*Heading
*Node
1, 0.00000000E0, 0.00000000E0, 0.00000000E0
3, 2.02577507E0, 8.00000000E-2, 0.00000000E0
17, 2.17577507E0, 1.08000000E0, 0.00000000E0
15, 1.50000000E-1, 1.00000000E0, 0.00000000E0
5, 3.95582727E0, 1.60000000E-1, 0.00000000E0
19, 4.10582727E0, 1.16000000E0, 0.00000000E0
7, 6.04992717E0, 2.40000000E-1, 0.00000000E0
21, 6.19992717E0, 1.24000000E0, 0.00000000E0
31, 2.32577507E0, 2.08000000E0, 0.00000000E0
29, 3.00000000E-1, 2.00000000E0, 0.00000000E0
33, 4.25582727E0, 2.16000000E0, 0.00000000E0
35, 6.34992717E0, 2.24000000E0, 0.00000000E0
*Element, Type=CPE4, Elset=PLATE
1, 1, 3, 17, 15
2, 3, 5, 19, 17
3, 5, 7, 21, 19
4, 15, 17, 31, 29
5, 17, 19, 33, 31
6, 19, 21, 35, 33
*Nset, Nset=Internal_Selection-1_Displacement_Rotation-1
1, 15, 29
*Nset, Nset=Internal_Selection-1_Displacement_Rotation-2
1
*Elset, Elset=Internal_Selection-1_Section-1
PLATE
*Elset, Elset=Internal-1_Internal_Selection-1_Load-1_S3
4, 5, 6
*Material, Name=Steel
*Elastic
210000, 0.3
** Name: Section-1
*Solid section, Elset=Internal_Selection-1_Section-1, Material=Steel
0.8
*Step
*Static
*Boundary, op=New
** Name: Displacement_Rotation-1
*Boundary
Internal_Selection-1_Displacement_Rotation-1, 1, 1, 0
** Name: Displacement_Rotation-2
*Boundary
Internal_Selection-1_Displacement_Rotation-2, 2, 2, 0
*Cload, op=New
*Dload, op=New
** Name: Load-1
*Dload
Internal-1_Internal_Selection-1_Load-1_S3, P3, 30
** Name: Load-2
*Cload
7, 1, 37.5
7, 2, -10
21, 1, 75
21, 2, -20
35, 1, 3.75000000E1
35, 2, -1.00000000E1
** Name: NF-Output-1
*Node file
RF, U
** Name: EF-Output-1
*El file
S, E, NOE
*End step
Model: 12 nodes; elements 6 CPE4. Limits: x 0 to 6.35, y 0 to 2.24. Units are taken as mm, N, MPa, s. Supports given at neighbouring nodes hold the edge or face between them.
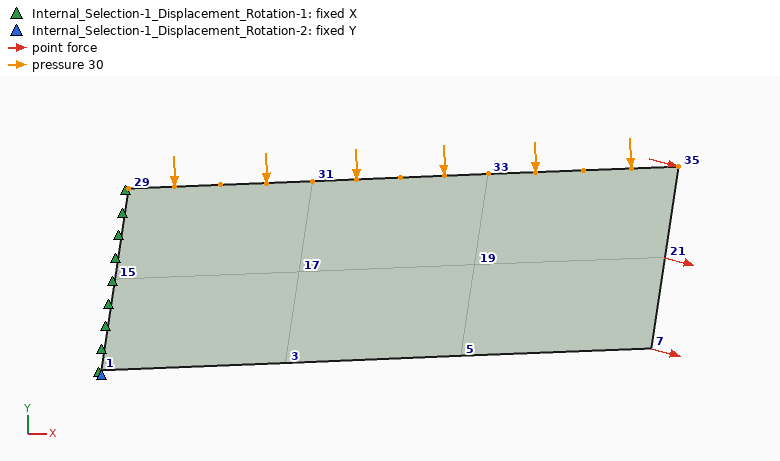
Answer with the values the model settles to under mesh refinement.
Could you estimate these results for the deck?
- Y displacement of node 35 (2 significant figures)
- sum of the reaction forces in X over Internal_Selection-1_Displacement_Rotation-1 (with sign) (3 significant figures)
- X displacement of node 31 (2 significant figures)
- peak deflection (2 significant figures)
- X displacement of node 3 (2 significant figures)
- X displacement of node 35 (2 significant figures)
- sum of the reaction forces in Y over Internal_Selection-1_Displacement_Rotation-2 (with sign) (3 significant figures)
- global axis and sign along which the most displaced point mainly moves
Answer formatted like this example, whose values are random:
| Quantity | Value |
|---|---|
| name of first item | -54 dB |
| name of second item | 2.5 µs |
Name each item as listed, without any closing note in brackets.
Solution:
| Quantity | Value |
|---|---|
| Y displacement of node 35 | -0.077 mm |
| sum of the reaction forces in X over Internal_Selection-1_Displacement_Rotation-1 (with sign) | -156 N |
| X displacement of node 31 | 0.011 mm |
| peak deflection | 0.080 mm |
| X displacement of node 3 | -0.0076 mm |
| X displacement of node 35 | 0.021 mm |
| sum of the reaction forces in Y over Internal_Selection-1_Displacement_Rotation-2 (with sign) | 185 N |
| global axis and sign along which the most displaced point mainly moves | -Y |
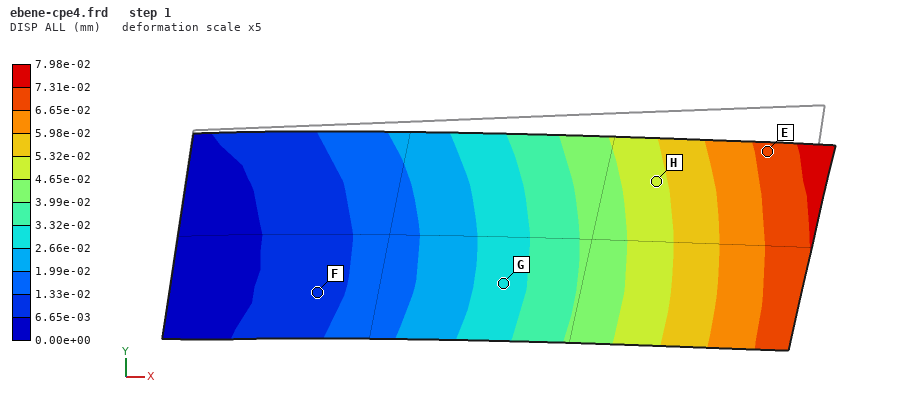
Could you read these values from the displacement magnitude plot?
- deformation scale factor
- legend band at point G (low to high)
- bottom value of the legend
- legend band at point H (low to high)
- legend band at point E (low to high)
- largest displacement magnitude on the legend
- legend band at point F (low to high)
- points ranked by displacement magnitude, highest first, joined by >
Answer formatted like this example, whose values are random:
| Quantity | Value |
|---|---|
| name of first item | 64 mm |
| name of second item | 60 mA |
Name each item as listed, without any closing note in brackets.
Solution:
| Quantity | Value |
|---|---|
| deformation scale factor | 5 |
| legend band at point G | 2.66e-02 to 3.32e-02 mm |
| bottom value of the legend | 0.00e+00 mm |
| legend band at point H | 4.65e-02 to 5.32e-02 mm |
| legend band at point E | 6.65e-02 to 7.31e-02 mm |
| largest displacement magnitude on the legend | 7.98e-02 mm |
| legend band at point F | 6.65e-03 to 1.33e-02 mm |
| points ranked by displacement magnitude, highest first, joined by > | E > H > G > F |
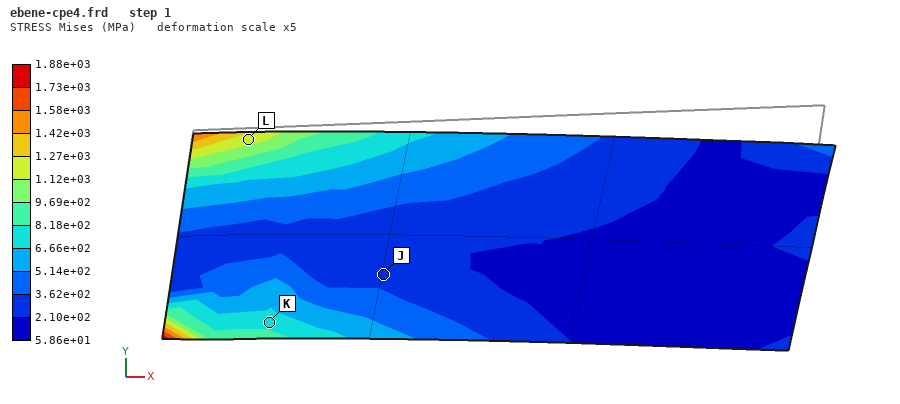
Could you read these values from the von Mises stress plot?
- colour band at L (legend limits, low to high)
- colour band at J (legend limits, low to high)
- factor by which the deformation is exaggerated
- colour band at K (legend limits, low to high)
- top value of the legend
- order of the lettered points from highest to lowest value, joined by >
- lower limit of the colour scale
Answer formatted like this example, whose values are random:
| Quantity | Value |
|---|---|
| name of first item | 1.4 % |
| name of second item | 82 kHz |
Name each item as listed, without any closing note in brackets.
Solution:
| Quantity | Value |
|---|---|
| colour band at L | 1.12e+03 to 1.27e+03 MPa |
| colour band at J | 2.10e+02 to 3.62e+02 MPa |
| factor by which the deformation is exaggerated | 5 |
| colour band at K | 6.66e+02 to 8.18e+02 MPa |
| top value of the legend | 1.88e+03 MPa |
| order of the lettered points from highest to lowest value, joined by > | L > K > J |
| lower limit of the colour scale | 5.86e+01 MPa |
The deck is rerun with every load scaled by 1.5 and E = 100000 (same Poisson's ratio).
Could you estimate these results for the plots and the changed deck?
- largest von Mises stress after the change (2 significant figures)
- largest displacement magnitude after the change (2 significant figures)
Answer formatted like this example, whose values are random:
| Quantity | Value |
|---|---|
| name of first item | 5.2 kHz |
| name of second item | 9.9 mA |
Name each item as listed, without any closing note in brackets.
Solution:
| Quantity | Value |
|---|---|
| largest von Mises stress after the change | 2800 MPa |
| largest displacement magnitude after the change | 0.25 mm |
